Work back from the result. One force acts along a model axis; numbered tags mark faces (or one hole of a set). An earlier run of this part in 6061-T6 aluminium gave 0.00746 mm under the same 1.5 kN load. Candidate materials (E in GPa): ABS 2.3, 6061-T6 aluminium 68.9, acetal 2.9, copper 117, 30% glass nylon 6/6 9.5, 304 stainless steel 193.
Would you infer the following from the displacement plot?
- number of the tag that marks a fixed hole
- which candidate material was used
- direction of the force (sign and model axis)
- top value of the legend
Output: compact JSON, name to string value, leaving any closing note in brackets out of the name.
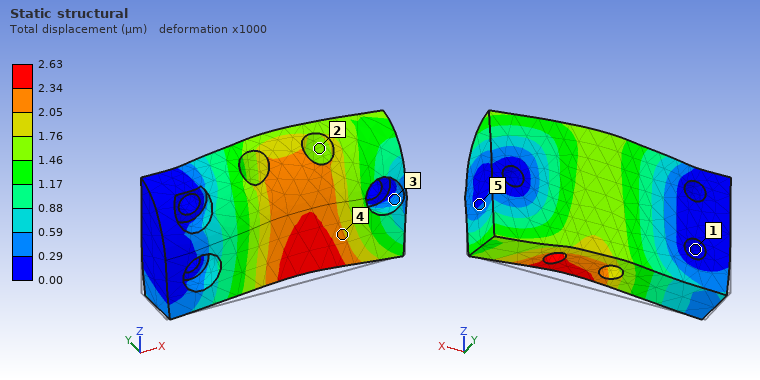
{"number of the tag that marks a fixed hole": "1", "which candidate material was used": "304 stainless steel", "direction of the force": "+Z", "top value of the legend": "2.63 µm"}
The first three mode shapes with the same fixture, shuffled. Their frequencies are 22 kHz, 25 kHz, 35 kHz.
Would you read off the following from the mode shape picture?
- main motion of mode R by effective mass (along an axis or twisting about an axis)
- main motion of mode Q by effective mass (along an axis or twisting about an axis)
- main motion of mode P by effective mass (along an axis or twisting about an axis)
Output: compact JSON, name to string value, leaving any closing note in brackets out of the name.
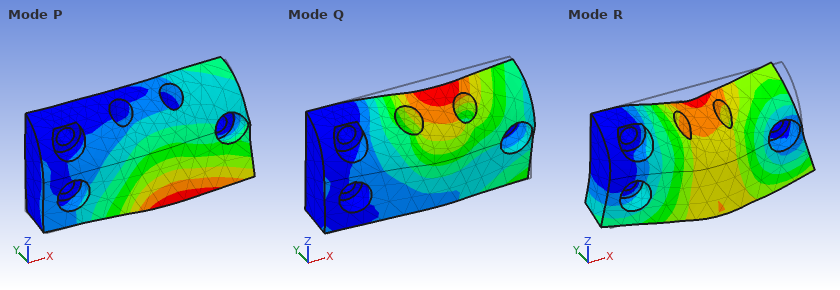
{"main motion of mode R by effective mass": "along Z", "main motion of mode Q by effective mass": "along Y", "main motion of mode P by effective mass": "along Y"}
